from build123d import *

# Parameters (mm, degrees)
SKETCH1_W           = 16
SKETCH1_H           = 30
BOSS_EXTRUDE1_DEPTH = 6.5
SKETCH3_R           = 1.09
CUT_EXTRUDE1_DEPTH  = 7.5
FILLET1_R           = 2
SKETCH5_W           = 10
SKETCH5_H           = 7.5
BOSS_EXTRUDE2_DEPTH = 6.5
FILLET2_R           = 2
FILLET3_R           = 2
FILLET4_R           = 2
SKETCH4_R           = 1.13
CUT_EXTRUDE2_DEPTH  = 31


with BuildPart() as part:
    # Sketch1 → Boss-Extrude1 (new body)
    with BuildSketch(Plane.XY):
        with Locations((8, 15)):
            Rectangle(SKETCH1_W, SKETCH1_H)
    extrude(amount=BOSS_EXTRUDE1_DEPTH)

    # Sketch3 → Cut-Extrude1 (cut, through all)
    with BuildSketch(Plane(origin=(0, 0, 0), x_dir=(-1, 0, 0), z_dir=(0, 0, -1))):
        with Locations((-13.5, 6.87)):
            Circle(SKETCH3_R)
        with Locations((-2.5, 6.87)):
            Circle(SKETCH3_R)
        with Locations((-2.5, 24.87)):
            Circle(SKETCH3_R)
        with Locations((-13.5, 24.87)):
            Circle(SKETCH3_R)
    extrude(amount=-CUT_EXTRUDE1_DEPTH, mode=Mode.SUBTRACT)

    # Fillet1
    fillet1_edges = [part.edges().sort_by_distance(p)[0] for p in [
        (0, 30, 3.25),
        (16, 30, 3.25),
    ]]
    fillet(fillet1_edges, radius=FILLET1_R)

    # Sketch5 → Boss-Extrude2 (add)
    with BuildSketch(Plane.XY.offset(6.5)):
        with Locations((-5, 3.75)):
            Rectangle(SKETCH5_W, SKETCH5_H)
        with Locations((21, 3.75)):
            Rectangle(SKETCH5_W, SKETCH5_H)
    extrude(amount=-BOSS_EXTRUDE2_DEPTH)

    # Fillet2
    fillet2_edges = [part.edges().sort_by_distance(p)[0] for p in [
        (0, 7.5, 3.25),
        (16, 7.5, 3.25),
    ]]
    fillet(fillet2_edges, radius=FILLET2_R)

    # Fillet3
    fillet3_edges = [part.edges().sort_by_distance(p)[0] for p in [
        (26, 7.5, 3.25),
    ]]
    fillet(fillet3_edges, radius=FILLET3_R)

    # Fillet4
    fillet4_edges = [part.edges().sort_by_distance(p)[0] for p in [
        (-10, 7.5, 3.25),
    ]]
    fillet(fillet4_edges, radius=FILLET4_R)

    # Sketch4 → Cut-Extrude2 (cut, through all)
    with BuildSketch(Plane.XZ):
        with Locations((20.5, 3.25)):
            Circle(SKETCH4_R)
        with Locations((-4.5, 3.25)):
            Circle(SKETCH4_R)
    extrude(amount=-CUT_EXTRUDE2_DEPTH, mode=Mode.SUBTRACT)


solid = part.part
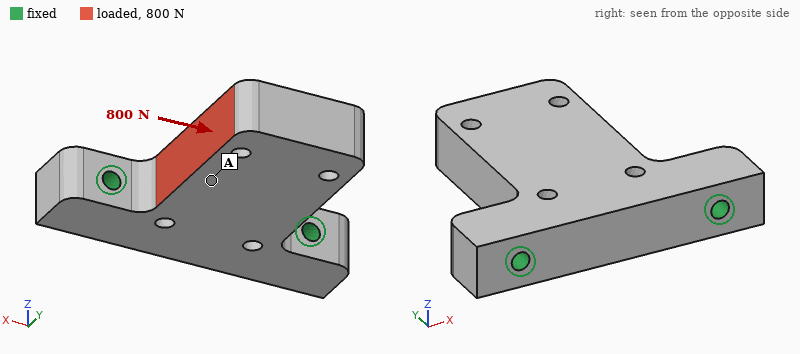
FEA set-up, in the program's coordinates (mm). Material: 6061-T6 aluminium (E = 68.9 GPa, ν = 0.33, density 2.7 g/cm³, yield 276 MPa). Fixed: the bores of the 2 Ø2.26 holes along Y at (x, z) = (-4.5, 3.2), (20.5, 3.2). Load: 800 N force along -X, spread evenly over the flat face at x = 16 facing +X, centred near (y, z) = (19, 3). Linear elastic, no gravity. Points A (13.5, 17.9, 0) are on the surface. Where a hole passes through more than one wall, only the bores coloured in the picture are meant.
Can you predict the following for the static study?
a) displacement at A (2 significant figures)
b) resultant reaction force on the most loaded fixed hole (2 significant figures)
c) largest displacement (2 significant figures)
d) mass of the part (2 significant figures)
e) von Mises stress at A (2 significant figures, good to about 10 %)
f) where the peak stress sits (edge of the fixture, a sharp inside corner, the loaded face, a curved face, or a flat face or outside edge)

11 µm
680 N
21 µm
11 g
12 MPa
a curved face
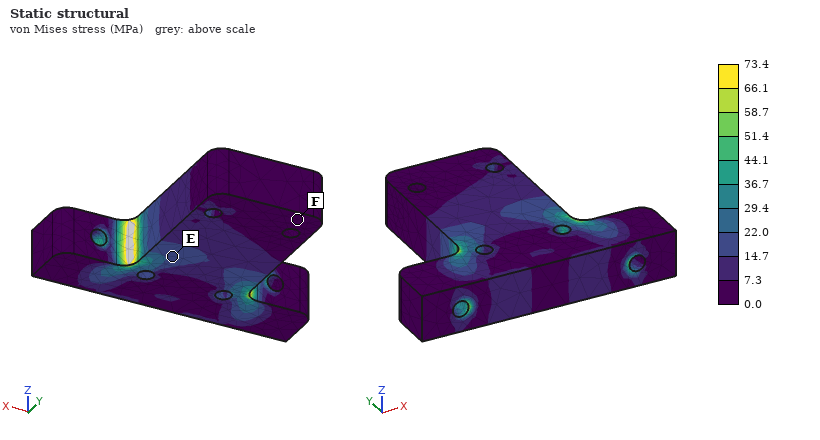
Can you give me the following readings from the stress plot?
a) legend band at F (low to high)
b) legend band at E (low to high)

0.0 to 7.3 MPa
14.7 to 22.0 MPa
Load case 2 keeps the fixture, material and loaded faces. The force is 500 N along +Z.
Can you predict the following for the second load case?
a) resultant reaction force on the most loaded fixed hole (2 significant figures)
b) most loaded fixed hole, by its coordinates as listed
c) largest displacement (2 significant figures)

440 N
(20.5, 3.2)
0.13 mm
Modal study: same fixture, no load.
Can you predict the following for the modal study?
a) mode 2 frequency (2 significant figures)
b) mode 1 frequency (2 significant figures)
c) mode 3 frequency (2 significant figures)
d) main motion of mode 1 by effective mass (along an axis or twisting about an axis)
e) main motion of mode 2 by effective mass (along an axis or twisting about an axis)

15 kHz
5200 Hz
21 kHz
along Z
along X
